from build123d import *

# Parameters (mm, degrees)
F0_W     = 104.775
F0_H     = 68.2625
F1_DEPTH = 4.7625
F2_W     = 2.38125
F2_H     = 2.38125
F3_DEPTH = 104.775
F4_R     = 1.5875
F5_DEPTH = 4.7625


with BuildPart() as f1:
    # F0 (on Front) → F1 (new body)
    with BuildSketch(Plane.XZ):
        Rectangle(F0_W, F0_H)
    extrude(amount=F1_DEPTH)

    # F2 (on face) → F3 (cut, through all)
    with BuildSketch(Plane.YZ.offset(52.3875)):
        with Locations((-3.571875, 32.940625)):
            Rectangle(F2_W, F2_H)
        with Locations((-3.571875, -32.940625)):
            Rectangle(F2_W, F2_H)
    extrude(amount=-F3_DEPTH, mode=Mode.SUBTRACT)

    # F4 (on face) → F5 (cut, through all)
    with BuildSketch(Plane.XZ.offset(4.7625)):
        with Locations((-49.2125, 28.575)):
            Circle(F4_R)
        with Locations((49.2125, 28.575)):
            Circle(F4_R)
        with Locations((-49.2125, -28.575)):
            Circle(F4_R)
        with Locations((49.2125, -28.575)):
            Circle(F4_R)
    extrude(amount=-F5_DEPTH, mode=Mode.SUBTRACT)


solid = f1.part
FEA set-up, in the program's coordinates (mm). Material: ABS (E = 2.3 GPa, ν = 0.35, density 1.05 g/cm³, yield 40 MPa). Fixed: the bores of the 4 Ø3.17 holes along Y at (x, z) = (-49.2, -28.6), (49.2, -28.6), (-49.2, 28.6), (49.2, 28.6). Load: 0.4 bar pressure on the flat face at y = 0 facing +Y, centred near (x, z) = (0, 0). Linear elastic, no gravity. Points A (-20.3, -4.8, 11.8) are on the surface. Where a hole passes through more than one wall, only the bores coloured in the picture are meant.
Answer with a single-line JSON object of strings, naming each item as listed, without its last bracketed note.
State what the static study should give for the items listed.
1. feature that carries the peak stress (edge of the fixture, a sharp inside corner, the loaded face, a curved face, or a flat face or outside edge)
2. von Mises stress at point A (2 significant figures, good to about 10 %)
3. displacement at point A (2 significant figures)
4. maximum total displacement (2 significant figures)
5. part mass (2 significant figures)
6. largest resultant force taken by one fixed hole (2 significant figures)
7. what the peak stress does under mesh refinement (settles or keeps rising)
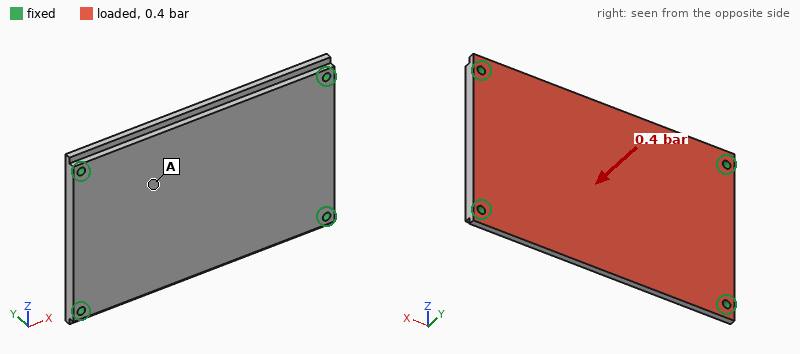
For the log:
{"feature that carries the peak stress": "edge of the fixture", "von Mises stress at point A": "3.5 MPa", "displacement at point A": "0.63 mm", "maximum total displacement": "0.84 mm", "part mass": "34 g", "largest resultant force taken by one fixed hole": "71 N", "what the peak stress does under mesh refinement": "keeps rising"}
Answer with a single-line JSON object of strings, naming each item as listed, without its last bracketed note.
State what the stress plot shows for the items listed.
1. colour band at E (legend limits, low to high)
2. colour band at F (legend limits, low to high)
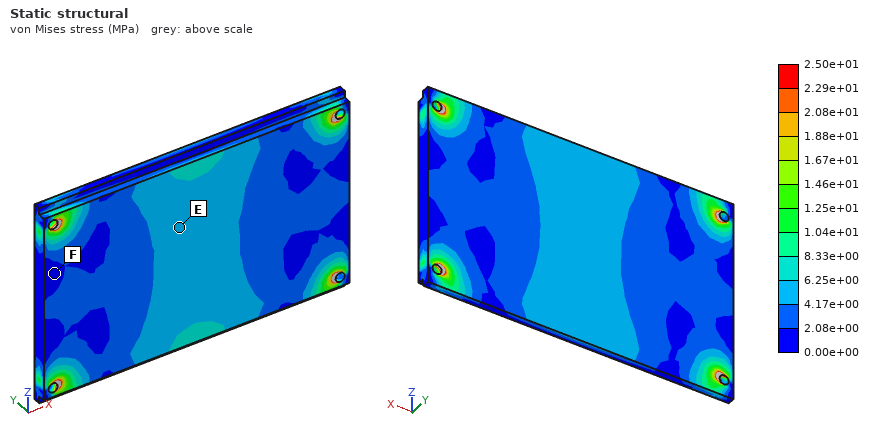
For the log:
{"colour band at E": "4.17e+00 to 6.25e+00 MPa", "colour band at F": "0.00e+00 to 2.08e+00 MPa"}
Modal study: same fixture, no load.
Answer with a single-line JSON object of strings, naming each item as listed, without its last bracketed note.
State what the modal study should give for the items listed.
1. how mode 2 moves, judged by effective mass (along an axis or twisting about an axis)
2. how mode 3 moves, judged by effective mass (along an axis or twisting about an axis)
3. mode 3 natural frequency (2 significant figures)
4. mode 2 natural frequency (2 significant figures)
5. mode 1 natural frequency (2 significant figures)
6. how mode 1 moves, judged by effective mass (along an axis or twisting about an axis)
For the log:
{"how mode 2 moves, judged by effective mass": "twisting about X", "how mode 3 moves, judged by effective mass": "twisting about Z", "mode 3 natural frequency": "1500 Hz", "mode 2 natural frequency": "970 Hz", "mode 1 natural frequency": "570 Hz", "how mode 1 moves, judged by effective mass": "along Y"}
